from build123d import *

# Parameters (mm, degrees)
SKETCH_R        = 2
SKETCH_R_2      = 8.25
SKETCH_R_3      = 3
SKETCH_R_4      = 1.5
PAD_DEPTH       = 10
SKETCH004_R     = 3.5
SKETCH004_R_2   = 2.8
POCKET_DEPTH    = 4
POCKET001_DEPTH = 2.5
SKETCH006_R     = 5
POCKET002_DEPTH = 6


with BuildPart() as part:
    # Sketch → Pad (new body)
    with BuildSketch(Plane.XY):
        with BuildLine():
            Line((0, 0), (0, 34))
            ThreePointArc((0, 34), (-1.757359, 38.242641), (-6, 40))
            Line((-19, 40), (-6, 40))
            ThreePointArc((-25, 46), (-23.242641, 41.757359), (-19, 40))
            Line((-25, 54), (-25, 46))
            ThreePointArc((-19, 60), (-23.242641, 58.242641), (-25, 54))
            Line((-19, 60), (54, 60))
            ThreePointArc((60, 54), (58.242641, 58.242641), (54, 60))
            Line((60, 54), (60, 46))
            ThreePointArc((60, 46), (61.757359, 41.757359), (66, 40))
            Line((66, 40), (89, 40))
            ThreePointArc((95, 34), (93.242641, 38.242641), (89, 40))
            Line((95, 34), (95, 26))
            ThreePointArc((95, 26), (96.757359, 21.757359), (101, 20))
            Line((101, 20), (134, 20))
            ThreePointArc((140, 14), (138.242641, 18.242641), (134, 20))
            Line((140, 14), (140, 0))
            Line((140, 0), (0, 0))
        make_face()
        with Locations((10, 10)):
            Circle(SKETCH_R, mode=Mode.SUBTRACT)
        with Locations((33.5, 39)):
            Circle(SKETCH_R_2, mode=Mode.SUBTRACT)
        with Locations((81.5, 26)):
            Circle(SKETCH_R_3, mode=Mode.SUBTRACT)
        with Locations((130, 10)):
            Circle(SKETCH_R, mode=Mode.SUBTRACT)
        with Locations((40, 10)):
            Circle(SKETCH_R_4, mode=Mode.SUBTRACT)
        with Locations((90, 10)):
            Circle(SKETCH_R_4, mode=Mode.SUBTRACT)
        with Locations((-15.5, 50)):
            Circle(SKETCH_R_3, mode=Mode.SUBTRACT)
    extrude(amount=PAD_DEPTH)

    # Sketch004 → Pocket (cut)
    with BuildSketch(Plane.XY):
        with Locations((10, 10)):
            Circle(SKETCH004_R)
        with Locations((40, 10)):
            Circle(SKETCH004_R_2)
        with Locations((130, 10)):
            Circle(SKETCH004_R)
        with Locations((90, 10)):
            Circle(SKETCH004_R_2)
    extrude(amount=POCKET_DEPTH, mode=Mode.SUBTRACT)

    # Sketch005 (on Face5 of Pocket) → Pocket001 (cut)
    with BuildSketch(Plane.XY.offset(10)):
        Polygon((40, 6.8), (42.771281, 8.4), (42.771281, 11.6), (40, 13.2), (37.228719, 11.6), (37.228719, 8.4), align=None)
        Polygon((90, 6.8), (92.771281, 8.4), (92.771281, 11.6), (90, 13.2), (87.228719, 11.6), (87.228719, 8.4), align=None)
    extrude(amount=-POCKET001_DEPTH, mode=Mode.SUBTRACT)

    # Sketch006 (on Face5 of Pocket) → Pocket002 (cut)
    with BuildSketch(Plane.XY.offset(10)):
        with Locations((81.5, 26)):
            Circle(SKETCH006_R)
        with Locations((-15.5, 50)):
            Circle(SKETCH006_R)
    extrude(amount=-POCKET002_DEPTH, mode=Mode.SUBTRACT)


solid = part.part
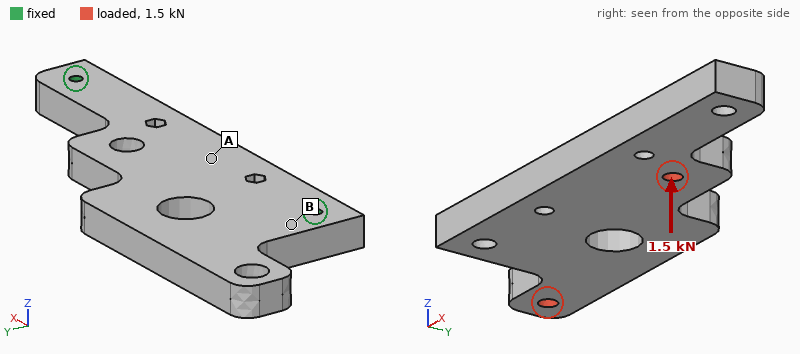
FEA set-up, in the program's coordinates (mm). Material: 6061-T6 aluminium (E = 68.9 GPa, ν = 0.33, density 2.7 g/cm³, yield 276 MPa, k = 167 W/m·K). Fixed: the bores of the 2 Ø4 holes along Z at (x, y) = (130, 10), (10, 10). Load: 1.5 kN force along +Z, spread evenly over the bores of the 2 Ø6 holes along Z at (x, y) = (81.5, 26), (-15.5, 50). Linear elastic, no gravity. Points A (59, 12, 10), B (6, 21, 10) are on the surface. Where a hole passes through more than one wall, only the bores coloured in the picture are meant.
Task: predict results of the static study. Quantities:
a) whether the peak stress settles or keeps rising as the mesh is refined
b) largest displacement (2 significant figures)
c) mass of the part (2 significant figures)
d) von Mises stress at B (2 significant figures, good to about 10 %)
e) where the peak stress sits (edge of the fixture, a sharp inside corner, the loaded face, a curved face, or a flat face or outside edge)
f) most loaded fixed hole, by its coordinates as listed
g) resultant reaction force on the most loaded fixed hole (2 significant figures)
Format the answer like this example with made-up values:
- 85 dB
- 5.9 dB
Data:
- keeps rising
- 0.39 mm
- 160 g
- 50 MPa
- edge of the fixture
- (10, 10)
- 1.2 kN
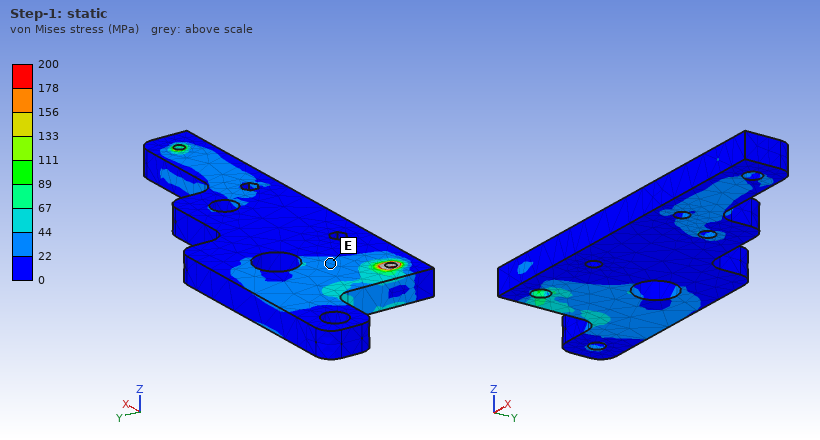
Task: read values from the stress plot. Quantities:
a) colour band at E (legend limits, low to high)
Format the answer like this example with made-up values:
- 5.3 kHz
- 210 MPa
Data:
- 22 to 44 MPa
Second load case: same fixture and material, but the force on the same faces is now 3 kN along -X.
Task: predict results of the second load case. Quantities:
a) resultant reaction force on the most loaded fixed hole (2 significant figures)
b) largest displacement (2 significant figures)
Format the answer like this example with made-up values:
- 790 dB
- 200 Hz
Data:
- 1.7 kN
- 60 µm
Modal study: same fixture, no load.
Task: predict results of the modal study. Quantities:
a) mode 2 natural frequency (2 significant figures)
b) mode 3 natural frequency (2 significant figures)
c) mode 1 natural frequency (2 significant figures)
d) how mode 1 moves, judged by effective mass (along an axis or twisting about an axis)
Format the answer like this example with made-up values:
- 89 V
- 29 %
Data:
- 2200 Hz
- 3800 Hz
- 1400 Hz
- along Z
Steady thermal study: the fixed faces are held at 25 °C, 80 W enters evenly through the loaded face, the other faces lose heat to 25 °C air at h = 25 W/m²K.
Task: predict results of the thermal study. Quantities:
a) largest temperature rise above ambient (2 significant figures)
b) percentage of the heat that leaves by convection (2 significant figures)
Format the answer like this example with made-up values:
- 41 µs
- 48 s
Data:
- 71 K
- 15 %
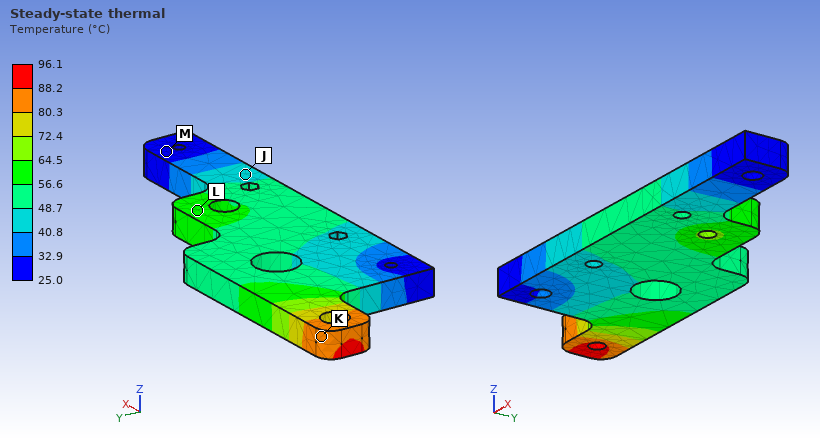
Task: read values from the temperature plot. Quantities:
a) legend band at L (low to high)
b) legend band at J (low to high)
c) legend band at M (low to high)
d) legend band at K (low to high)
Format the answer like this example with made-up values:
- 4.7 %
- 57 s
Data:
- 56.6 to 64.5 °C
- 40.8 to 48.7 °C
- 25.0 to 32.9 °C
- 80.3 to 88.2 °C
